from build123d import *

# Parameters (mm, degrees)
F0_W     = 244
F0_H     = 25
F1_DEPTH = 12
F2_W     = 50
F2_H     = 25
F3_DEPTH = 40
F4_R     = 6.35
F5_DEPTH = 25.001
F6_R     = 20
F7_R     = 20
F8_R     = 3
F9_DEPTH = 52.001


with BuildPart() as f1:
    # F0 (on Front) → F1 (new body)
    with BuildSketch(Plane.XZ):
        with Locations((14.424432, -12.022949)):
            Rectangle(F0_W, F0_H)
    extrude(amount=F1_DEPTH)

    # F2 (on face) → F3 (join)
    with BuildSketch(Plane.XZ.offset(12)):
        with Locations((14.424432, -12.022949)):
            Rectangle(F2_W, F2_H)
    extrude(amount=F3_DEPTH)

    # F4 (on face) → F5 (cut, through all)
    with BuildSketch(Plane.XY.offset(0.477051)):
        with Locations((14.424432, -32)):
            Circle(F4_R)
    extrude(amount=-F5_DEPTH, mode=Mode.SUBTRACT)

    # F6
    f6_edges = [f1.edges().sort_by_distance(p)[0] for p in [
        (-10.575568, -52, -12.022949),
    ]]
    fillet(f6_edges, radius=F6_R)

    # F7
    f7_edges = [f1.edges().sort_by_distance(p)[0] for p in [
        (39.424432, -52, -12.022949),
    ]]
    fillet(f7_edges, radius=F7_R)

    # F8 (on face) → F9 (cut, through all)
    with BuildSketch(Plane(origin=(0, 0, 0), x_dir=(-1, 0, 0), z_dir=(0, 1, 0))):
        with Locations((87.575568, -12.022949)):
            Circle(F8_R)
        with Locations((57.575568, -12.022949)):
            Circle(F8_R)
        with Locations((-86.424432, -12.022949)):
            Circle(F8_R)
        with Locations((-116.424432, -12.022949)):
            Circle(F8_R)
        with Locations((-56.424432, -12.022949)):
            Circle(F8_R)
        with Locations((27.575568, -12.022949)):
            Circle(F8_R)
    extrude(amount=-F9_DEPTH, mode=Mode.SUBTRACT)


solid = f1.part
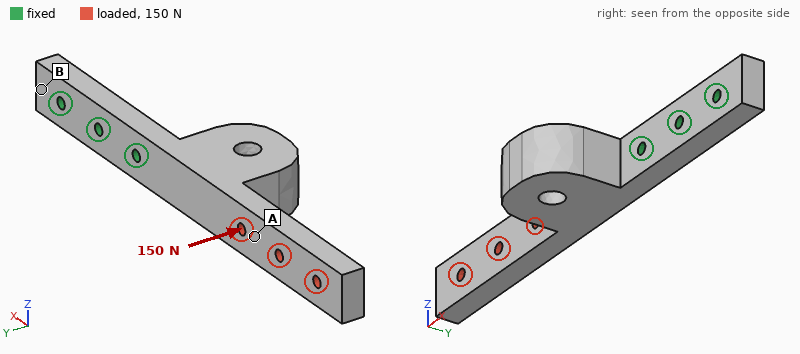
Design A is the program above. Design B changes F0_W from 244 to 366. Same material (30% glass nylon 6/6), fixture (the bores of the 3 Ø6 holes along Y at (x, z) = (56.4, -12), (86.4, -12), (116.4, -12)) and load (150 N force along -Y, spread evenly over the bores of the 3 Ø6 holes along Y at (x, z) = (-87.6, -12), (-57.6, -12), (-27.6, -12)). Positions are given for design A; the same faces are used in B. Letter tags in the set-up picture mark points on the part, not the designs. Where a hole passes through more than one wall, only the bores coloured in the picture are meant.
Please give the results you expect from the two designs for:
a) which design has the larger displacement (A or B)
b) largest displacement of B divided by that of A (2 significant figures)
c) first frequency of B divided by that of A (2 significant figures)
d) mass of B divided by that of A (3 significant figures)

B
1.5
0.54
1.32
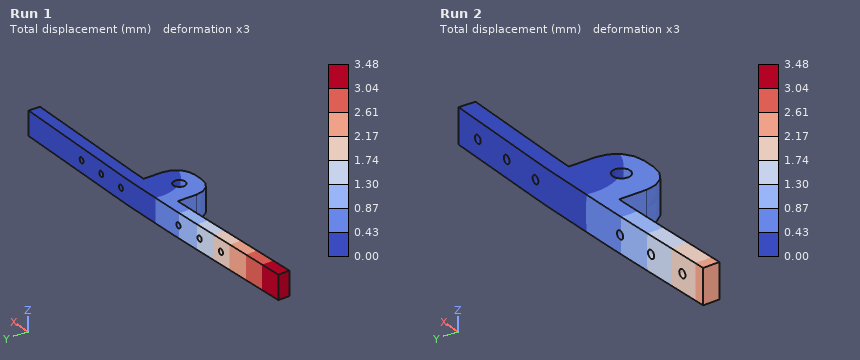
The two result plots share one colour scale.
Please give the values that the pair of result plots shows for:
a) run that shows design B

Run 1
